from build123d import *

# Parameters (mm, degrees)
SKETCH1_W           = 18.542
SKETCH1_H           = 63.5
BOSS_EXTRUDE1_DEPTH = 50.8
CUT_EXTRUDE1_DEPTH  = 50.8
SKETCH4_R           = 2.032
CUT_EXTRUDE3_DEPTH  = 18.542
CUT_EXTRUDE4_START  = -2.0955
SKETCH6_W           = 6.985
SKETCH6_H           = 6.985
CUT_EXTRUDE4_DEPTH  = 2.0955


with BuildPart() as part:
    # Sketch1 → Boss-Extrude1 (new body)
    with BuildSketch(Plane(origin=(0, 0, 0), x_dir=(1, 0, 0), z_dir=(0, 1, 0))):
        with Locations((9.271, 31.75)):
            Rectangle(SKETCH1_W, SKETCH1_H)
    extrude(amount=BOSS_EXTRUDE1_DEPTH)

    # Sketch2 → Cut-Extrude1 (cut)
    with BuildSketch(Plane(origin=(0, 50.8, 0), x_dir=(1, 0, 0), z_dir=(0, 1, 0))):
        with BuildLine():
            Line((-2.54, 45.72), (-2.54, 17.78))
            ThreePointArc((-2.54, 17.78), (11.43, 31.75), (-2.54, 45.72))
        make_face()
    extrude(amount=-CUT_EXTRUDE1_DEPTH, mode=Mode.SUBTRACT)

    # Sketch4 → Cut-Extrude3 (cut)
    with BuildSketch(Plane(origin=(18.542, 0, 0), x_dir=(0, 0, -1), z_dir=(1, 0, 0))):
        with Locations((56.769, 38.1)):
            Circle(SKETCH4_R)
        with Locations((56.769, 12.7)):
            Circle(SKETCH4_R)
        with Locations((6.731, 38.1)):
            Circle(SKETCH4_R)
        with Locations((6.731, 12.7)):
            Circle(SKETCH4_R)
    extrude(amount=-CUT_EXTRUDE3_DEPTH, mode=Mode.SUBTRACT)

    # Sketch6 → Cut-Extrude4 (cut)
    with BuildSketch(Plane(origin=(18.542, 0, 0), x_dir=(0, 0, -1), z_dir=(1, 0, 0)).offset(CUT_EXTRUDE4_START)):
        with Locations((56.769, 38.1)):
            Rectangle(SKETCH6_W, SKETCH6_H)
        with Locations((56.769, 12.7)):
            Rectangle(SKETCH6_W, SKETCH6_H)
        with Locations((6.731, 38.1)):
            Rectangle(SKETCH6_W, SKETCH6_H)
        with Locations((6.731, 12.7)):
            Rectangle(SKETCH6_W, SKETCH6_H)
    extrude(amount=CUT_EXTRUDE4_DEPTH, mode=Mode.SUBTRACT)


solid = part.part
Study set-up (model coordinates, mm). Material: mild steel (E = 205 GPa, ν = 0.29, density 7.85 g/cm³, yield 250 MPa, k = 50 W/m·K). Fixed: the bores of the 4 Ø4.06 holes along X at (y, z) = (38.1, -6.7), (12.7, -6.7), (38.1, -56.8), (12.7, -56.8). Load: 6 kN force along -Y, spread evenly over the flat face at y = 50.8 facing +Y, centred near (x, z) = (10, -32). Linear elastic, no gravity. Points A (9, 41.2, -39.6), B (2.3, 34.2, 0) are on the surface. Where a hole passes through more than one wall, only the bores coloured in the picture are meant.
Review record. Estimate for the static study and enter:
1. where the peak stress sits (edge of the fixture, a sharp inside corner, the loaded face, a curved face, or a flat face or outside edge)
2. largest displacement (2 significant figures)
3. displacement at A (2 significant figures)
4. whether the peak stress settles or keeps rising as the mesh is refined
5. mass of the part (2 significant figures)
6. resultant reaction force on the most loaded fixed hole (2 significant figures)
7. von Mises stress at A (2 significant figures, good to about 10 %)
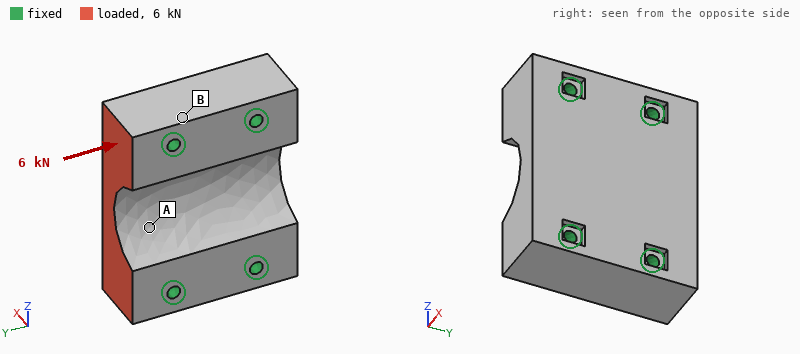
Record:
edge of the fixture
1.4 µm
0.81 µm
keeps rising
370 g
2.3 kN
5.0 MPa
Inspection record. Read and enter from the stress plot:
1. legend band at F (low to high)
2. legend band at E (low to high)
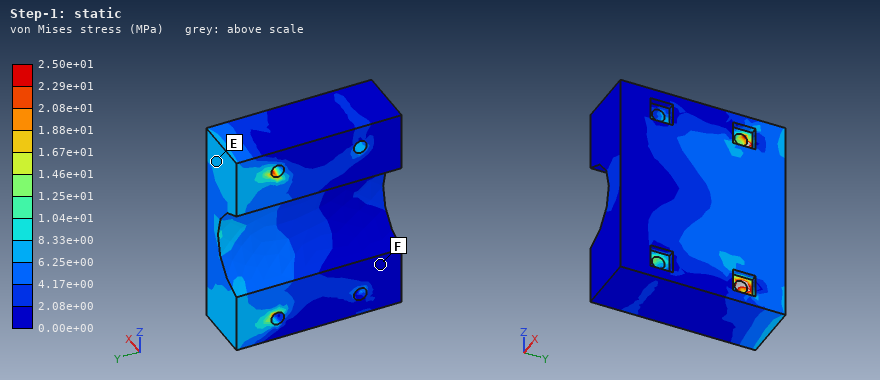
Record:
0.00e+00 to 2.08e+00 MPa
6.25e+00 to 8.33e+00 MPa
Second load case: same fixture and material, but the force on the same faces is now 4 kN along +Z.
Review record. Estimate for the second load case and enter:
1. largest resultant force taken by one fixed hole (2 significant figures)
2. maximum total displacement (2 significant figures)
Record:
2.1 kN
1.9 µm
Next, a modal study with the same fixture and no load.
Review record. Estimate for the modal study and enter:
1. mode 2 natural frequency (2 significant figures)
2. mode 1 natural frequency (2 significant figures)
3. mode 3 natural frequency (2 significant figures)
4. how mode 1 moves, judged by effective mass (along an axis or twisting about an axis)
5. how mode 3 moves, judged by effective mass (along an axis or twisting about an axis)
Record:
23 kHz
22 kHz
30 kHz
along X
along Y
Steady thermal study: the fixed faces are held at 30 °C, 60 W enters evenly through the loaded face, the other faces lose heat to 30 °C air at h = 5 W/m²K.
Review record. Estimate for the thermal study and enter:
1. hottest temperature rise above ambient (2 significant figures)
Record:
26 K
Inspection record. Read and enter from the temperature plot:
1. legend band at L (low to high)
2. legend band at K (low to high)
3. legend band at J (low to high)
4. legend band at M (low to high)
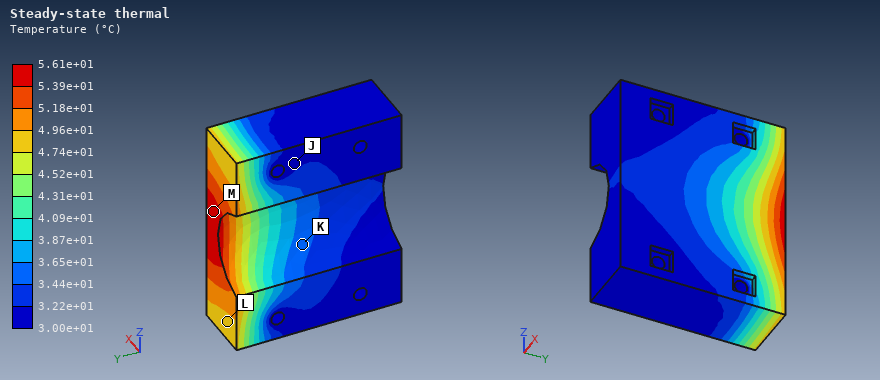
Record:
4.74e+01 to 4.96e+01 °C
3.44e+01 to 3.65e+01 °C
3.00e+01 to 3.22e+01 °C
5.39e+01 to 5.61e+01 °C
